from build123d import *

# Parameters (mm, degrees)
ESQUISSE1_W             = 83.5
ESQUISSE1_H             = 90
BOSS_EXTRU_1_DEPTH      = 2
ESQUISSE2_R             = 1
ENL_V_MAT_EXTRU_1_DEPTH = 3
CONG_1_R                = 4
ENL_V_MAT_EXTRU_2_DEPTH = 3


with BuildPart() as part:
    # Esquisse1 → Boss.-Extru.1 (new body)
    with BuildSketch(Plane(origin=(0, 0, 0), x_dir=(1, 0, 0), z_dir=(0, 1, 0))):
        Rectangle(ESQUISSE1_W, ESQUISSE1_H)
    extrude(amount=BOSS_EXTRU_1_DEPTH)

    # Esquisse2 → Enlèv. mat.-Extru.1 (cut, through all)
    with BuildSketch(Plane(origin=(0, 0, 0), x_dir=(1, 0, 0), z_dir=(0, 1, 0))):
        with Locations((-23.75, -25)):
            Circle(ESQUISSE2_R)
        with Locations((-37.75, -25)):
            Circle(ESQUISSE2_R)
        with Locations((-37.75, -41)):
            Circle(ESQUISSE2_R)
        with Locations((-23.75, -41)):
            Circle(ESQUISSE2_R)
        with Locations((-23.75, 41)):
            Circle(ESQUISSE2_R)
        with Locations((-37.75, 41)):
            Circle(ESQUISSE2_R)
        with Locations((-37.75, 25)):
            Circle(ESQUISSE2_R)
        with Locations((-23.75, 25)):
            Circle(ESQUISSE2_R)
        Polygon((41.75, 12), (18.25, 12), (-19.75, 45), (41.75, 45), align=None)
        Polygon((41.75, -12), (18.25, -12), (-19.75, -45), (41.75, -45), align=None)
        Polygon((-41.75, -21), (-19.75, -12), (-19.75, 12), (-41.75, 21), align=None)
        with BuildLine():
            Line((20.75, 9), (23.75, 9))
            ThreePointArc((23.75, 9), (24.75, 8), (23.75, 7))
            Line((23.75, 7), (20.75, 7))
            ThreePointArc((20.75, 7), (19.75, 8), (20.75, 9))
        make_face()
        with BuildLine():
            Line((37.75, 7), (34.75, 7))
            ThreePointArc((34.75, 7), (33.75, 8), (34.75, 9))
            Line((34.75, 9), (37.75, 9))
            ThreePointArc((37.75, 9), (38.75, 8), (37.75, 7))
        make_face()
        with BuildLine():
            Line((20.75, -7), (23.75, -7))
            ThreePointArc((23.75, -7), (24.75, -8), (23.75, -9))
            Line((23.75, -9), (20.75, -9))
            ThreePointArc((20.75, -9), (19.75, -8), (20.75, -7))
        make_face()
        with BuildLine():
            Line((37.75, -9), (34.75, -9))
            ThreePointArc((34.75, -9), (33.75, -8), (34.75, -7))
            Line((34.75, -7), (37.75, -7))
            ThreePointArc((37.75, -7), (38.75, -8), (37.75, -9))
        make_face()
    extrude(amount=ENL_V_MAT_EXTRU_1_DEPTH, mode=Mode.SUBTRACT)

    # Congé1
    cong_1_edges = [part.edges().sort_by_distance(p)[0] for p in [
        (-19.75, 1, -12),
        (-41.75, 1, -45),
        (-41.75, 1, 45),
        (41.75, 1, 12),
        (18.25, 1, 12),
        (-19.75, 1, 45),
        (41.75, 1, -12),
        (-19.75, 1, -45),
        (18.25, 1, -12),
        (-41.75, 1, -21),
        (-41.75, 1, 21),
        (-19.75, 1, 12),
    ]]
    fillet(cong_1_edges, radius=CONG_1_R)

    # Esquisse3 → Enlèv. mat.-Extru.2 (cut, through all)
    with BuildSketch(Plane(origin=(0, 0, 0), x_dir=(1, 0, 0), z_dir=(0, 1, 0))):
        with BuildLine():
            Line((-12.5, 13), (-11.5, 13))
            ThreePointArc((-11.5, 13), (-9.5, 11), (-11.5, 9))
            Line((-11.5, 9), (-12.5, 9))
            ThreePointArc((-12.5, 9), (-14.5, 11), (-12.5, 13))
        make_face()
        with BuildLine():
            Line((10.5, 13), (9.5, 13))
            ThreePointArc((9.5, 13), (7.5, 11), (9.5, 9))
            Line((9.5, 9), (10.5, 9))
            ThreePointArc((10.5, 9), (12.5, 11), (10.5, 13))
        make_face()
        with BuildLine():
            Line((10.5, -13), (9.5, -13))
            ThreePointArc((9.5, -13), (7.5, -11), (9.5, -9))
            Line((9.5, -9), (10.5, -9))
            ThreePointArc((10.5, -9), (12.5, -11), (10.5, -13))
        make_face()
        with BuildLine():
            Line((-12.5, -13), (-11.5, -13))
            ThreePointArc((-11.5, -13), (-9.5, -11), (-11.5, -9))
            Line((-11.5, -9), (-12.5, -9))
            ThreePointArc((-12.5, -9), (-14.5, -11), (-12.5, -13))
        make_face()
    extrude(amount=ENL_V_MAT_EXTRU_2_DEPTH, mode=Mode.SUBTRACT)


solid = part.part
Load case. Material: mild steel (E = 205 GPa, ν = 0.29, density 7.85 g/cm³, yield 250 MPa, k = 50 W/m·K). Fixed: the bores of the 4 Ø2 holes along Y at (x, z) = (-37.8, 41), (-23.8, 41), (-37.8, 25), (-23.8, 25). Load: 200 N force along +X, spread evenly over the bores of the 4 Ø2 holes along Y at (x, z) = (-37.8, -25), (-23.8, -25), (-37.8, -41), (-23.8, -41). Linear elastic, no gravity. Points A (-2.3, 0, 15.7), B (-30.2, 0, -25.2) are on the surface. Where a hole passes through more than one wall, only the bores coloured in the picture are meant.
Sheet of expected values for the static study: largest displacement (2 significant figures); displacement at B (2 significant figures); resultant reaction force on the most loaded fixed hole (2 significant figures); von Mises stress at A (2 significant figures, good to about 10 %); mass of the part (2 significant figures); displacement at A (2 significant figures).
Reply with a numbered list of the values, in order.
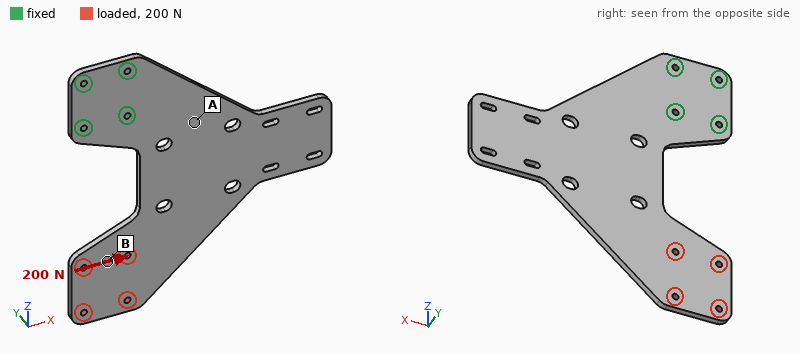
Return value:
1. 51 µm
2. 34 µm
3. 480 N
4. 17 MPa
5. 60 g
6. 9.2 µm
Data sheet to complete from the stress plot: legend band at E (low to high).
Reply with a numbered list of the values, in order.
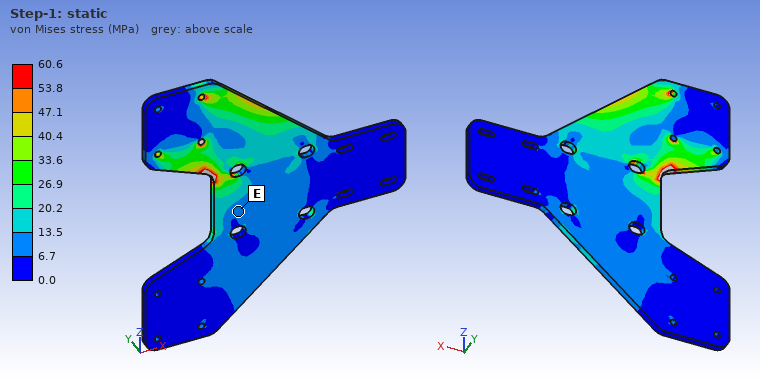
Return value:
1. 6.7 to 13.5 MPa
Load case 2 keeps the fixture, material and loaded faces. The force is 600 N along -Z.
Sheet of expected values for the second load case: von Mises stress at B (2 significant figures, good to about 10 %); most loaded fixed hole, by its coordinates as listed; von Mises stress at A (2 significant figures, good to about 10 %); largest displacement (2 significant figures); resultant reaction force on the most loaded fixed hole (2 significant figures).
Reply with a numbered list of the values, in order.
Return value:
1. 19 MPa
2. (-23.8, 25)
3. 12 MPa
4. 62 µm
5. 470 N
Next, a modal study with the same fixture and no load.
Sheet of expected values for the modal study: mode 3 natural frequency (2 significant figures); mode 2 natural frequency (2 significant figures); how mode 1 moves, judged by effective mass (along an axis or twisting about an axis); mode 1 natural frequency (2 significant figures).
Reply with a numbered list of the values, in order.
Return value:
1. 1400 Hz
2. 360 Hz
3. along Y
4. 260 Hz
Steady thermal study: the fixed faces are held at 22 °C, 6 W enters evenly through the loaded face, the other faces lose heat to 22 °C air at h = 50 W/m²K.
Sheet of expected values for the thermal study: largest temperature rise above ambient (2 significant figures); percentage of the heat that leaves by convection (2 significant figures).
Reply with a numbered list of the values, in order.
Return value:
1. 52 K
2. 92 %
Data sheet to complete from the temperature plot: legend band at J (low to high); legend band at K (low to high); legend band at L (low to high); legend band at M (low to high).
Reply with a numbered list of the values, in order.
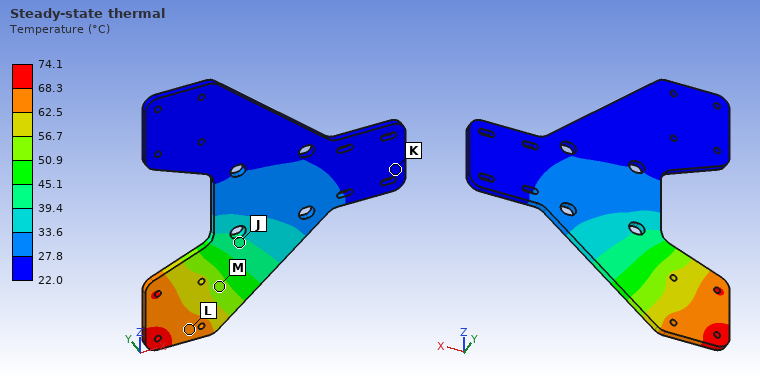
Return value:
1. 39.4 to 45.1 °C
2. 22.0 to 27.8 °C
3. 62.5 to 68.3 °C
4. 50.9 to 56.7 °C
